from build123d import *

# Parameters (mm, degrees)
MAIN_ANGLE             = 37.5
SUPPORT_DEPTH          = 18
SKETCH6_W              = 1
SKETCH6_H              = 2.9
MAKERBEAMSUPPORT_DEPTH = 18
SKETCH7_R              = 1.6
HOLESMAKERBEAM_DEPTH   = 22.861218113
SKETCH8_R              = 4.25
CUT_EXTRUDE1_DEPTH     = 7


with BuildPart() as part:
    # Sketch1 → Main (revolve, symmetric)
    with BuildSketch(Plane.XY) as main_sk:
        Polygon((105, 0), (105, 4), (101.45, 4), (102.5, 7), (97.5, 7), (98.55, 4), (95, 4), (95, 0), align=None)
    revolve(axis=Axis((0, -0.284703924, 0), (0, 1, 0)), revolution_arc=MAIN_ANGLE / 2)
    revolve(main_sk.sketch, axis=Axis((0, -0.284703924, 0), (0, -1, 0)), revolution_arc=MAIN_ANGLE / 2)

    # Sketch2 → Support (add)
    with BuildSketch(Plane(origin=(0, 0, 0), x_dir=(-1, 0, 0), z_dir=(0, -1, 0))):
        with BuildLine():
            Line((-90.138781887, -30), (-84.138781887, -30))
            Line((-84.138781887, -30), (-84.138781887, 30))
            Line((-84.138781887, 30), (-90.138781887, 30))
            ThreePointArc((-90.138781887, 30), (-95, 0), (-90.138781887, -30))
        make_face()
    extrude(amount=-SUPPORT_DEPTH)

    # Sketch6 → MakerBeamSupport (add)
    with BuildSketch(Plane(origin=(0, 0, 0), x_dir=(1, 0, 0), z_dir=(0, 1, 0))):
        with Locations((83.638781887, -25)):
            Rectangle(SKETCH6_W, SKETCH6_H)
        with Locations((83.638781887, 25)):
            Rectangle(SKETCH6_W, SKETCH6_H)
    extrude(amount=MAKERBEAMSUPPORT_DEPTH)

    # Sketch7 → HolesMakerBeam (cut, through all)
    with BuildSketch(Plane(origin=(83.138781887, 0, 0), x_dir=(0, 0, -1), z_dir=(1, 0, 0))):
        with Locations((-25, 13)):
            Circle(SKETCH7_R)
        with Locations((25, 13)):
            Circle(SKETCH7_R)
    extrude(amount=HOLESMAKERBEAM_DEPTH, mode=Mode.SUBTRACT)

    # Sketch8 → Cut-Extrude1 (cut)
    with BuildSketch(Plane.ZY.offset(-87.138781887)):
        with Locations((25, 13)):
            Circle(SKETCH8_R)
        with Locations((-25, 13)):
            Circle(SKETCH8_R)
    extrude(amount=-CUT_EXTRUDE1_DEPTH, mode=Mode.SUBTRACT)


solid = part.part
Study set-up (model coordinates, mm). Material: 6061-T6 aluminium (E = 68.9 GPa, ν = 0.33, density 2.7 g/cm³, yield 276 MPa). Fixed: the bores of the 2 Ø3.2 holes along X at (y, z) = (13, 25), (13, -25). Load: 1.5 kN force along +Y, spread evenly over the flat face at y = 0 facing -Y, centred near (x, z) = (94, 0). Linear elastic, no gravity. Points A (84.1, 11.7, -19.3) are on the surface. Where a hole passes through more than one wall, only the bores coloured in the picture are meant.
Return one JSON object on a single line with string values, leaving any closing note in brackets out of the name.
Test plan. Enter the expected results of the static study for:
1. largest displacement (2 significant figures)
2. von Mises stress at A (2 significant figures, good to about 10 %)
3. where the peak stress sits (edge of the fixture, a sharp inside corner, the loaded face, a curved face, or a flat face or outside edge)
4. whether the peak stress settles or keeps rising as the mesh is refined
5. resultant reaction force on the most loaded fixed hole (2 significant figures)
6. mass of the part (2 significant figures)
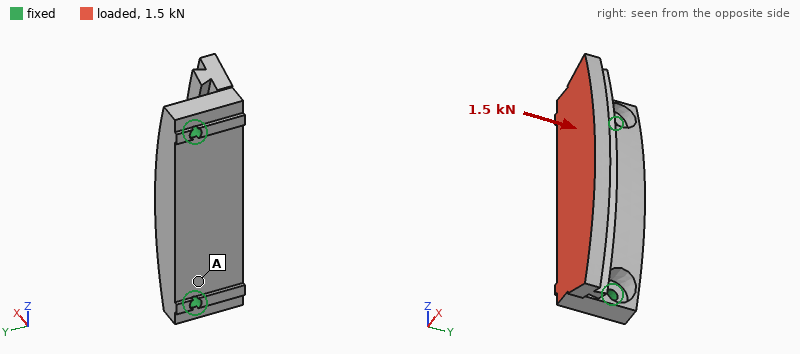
{"largest displacement": "0.11 mm", "von Mises stress at A": "26 MPa", "where the peak stress sits": "edge of the fixture", "whether the peak stress settles or keeps rising as the mesh is refined": "keeps rising", "resultant reaction force on the most loaded fixed hole": "810 N", "mass of the part": "35 g"}
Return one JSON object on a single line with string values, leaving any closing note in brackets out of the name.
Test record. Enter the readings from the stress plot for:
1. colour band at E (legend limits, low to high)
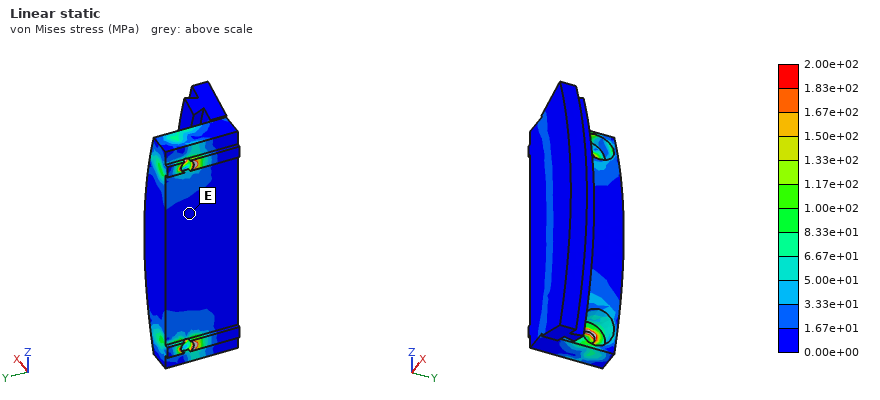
{"colour band at E": "0.00e+00 to 1.67e+01 MPa"}
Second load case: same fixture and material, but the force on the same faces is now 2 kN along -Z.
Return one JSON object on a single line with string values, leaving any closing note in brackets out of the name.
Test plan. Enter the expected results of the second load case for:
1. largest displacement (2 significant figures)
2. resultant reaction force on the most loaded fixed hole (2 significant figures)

{"largest displacement": "11 µm", "resultant reaction force on the most loaded fixed hole": "1.2 kN"}
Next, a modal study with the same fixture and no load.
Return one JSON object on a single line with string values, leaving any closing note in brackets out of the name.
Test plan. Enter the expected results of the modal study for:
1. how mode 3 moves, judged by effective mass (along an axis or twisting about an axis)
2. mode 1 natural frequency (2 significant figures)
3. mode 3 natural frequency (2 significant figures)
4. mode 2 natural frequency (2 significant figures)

{"how mode 3 moves, judged by effective mass": "along X", "mode 1 natural frequency": "4400 Hz", "mode 3 natural frequency": "12 kHz", "mode 2 natural frequency": "11 kHz"}
